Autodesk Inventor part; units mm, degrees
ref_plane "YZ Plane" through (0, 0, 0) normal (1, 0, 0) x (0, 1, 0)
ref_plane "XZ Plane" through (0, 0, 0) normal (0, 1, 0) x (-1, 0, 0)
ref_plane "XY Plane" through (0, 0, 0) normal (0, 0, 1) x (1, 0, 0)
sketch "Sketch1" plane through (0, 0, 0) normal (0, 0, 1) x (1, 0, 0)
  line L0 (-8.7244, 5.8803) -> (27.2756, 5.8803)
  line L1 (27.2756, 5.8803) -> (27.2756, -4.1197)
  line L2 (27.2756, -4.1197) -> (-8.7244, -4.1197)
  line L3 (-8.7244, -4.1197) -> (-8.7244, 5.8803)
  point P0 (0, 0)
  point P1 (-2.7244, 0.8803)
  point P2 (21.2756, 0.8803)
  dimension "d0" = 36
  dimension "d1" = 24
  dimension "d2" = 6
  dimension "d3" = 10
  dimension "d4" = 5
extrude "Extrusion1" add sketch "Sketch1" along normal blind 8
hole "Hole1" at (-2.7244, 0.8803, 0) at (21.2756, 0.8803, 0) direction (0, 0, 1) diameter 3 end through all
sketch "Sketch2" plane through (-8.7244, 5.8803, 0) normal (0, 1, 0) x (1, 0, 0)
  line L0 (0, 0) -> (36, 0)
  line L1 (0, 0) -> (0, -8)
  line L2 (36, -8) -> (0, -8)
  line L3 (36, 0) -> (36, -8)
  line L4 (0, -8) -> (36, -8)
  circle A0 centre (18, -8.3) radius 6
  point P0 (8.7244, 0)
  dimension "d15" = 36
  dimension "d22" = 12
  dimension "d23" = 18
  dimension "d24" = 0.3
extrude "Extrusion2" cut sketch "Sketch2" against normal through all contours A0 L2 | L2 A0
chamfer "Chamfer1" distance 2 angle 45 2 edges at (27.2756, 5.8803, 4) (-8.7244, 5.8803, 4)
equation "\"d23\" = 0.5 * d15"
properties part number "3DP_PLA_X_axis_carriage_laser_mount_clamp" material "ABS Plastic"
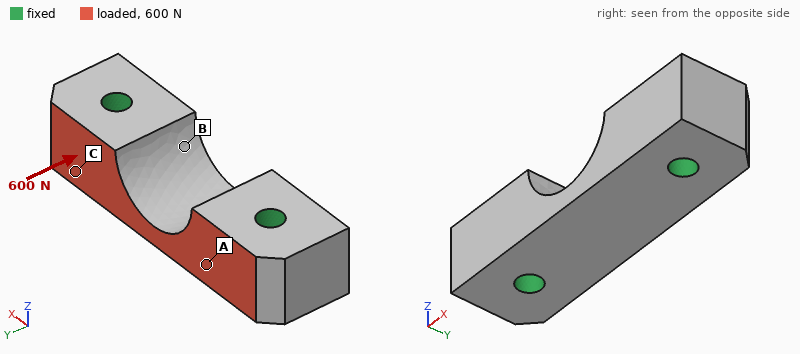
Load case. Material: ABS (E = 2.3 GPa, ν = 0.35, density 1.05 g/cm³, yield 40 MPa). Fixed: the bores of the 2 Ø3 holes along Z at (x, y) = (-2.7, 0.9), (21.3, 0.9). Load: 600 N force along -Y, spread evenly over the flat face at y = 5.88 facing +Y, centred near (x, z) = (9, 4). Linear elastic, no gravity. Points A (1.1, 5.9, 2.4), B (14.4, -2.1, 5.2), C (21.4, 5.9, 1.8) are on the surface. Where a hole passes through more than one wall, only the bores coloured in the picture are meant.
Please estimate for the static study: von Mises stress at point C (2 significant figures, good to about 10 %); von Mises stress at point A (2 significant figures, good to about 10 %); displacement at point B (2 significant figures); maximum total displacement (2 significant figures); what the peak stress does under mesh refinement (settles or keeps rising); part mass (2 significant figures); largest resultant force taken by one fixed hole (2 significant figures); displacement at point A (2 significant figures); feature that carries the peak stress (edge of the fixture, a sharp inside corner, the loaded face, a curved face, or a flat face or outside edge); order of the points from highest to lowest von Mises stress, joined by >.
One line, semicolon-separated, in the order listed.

5.3 MPa; 3.1 MPa; 27 µm; 55 µm; keeps rising; 2.3 g; 300 N; 27 µm; edge of the fixture; C > A > B
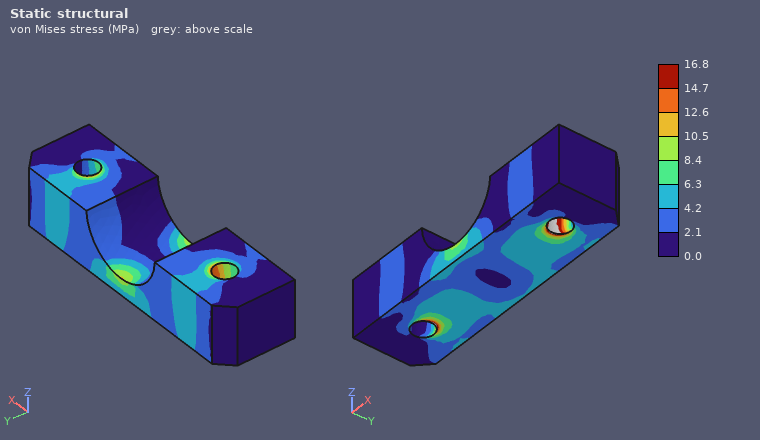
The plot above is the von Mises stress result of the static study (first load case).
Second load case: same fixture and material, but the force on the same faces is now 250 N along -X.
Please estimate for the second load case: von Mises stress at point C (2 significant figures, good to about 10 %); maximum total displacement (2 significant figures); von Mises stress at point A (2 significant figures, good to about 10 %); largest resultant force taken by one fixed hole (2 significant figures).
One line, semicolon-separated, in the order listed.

2.2 MPa; 17 µm; 2.4 MPa; 130 N
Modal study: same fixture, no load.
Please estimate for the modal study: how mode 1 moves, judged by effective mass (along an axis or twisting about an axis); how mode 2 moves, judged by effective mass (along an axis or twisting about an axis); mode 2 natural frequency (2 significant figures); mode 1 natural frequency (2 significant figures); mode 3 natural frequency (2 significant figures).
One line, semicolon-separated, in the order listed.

along Y; along Z; 17 kHz; 13 kHz; 21 kHz
